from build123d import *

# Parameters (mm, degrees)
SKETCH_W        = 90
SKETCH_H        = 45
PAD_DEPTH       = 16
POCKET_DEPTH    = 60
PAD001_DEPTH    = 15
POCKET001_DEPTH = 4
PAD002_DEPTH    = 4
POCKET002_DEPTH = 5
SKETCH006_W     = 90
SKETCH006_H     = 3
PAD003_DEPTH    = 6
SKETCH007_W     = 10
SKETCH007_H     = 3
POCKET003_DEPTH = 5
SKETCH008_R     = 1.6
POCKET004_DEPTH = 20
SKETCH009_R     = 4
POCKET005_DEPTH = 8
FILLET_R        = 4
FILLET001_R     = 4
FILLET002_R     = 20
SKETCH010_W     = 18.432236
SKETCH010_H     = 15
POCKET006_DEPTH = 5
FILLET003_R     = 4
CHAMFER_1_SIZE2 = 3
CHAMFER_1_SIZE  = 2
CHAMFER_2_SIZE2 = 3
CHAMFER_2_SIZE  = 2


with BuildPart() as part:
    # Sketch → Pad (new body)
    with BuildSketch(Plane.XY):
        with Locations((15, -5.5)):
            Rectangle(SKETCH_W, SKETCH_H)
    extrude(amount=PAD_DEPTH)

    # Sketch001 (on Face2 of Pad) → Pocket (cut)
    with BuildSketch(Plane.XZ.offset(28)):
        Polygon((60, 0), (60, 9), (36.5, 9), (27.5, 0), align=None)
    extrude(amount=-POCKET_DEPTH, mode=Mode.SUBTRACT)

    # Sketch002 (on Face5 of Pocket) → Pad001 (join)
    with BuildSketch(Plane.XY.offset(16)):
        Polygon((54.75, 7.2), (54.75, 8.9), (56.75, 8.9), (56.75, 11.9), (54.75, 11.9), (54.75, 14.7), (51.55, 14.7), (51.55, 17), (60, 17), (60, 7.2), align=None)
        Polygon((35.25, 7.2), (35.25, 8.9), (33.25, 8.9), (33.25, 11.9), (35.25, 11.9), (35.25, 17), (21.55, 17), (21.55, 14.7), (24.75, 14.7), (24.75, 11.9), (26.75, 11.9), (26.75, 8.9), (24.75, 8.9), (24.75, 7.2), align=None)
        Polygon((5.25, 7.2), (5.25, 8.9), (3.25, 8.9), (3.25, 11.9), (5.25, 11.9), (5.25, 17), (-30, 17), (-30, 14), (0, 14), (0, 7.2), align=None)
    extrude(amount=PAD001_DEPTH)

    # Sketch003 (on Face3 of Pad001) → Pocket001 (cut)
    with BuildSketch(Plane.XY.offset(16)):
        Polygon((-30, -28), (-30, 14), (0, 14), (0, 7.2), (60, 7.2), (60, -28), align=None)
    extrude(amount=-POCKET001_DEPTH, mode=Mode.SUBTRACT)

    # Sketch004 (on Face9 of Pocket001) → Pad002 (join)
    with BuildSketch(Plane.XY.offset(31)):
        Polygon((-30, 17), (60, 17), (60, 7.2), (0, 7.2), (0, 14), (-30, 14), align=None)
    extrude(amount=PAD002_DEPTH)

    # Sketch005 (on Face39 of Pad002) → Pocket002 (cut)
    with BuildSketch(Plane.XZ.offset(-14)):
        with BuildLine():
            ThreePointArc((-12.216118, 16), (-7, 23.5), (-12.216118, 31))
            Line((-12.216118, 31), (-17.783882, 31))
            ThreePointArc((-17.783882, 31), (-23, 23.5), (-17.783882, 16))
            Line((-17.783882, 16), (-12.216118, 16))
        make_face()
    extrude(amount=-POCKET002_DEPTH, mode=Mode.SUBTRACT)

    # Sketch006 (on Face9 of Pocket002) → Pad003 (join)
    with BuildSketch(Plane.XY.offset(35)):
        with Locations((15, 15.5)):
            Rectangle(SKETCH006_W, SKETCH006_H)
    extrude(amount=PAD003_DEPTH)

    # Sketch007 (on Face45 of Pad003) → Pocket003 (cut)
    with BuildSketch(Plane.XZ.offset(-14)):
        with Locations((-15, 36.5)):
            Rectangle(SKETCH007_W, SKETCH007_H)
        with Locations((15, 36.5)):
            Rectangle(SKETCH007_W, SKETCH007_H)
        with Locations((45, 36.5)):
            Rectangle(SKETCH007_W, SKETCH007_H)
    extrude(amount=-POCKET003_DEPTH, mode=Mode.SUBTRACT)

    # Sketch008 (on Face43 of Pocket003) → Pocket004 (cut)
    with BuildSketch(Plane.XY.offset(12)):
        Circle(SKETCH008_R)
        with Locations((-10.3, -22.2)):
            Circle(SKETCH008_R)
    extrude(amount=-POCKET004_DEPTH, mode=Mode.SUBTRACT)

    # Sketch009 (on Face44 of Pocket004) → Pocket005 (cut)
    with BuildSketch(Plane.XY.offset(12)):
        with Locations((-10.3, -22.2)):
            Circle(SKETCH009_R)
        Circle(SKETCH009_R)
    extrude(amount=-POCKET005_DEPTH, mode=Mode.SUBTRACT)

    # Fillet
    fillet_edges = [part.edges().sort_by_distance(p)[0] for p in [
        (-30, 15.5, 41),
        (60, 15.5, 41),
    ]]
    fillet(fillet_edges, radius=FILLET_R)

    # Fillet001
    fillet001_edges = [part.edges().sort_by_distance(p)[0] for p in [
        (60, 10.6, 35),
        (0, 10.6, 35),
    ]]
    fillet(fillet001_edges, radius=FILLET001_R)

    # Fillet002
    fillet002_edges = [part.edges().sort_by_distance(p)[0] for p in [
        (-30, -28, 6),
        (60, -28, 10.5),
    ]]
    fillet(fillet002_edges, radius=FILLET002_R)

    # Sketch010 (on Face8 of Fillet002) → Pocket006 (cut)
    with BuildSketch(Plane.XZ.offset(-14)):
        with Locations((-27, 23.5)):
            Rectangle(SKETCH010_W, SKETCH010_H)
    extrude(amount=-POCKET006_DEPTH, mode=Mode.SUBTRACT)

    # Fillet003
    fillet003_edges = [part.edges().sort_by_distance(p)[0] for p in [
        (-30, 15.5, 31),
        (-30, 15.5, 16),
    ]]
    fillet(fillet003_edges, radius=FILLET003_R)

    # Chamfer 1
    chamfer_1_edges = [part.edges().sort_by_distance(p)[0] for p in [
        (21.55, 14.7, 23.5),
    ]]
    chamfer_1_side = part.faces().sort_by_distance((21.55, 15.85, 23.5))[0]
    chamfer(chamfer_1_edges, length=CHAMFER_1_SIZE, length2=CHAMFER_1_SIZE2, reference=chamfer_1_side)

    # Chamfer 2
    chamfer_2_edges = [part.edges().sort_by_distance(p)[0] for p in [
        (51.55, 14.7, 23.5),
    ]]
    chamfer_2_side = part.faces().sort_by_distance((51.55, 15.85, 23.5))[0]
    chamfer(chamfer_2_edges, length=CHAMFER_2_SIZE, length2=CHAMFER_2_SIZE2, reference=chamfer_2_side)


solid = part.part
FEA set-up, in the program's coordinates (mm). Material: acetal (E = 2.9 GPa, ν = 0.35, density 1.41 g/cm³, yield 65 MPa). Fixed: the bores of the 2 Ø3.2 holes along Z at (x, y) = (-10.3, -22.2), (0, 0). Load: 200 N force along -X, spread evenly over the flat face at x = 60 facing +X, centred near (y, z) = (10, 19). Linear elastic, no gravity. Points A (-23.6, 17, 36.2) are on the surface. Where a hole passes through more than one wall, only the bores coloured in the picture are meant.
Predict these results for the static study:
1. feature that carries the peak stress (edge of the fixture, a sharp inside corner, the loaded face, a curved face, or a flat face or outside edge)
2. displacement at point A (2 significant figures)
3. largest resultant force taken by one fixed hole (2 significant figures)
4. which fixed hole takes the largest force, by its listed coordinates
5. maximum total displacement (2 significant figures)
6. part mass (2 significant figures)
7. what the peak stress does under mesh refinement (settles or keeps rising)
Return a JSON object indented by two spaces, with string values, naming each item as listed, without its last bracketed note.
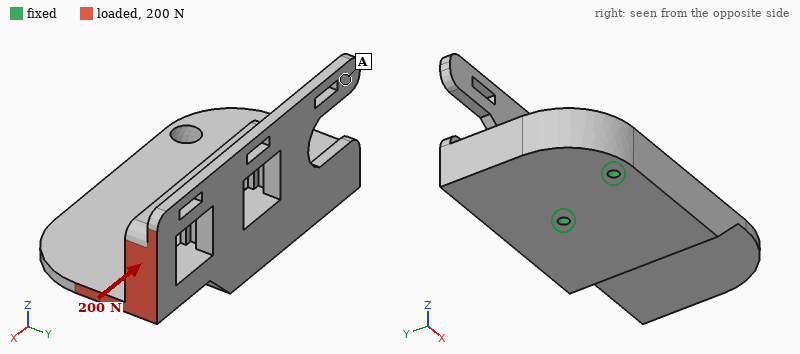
{
  "feature that carries the peak stress": "edge of the fixture",
  "displacement at point A": "0.73 mm",
  "largest resultant force taken by one fixed hole": "260 N",
  "which fixed hole takes the largest force, by its listed coordinates": "(0, 0)",
  "maximum total displacement": "1.1 mm",
  "part mass": "63 g",
  "what the peak stress does under mesh refinement": "keeps rising"
}
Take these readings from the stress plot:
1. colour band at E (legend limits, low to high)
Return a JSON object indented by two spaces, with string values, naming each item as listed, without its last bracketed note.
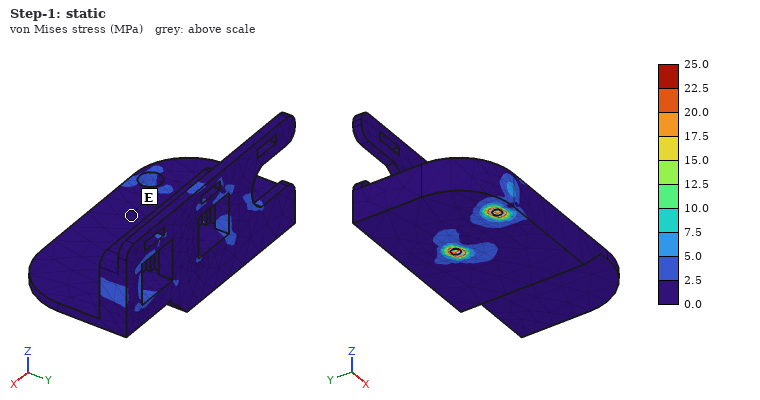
{
  "colour band at E": "0.0 to 2.5 MPa"
}
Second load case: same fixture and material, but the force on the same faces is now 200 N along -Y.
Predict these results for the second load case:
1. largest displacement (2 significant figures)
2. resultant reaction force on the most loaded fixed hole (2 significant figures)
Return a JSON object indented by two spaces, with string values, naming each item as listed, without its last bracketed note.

{
  "largest displacement": "1.1 mm",
  "resultant reaction force on the most loaded fixed hole": "560 N"
}
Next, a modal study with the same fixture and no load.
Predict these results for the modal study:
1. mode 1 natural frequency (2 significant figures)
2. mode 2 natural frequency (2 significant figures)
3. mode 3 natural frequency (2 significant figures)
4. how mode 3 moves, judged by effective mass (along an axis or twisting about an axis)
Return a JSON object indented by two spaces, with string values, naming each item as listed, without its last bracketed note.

{
  "mode 1 natural frequency": "350 Hz",
  "mode 2 natural frequency": "740 Hz",
  "mode 3 natural frequency": "870 Hz",
  "how mode 3 moves, judged by effective mass": "along Y"
}
